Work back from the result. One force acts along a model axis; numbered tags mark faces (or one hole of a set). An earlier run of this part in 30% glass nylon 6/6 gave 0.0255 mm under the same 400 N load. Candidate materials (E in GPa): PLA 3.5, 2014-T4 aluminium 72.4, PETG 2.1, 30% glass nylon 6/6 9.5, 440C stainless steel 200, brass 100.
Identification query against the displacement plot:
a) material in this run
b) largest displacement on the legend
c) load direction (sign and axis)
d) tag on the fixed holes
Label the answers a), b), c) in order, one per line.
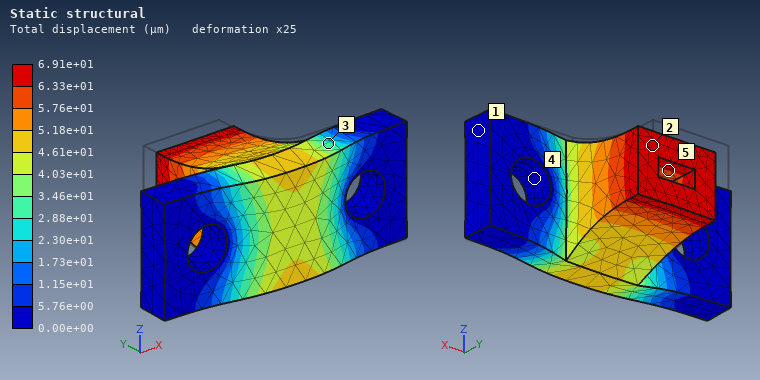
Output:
a) PLA
b) 6.91e+01 µm
c) -Y
d) 4
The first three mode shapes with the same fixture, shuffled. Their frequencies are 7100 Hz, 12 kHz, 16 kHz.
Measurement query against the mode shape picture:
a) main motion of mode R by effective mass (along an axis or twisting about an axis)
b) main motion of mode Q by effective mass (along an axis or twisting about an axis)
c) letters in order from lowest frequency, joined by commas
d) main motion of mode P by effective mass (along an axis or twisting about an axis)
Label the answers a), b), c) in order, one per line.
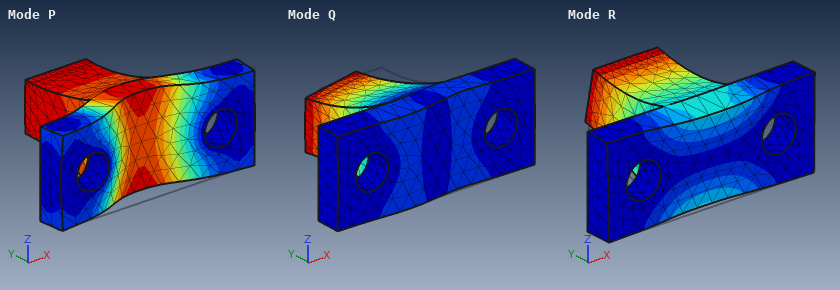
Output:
a) along Z
b) along X
c) R, Q, P
d) along Y
